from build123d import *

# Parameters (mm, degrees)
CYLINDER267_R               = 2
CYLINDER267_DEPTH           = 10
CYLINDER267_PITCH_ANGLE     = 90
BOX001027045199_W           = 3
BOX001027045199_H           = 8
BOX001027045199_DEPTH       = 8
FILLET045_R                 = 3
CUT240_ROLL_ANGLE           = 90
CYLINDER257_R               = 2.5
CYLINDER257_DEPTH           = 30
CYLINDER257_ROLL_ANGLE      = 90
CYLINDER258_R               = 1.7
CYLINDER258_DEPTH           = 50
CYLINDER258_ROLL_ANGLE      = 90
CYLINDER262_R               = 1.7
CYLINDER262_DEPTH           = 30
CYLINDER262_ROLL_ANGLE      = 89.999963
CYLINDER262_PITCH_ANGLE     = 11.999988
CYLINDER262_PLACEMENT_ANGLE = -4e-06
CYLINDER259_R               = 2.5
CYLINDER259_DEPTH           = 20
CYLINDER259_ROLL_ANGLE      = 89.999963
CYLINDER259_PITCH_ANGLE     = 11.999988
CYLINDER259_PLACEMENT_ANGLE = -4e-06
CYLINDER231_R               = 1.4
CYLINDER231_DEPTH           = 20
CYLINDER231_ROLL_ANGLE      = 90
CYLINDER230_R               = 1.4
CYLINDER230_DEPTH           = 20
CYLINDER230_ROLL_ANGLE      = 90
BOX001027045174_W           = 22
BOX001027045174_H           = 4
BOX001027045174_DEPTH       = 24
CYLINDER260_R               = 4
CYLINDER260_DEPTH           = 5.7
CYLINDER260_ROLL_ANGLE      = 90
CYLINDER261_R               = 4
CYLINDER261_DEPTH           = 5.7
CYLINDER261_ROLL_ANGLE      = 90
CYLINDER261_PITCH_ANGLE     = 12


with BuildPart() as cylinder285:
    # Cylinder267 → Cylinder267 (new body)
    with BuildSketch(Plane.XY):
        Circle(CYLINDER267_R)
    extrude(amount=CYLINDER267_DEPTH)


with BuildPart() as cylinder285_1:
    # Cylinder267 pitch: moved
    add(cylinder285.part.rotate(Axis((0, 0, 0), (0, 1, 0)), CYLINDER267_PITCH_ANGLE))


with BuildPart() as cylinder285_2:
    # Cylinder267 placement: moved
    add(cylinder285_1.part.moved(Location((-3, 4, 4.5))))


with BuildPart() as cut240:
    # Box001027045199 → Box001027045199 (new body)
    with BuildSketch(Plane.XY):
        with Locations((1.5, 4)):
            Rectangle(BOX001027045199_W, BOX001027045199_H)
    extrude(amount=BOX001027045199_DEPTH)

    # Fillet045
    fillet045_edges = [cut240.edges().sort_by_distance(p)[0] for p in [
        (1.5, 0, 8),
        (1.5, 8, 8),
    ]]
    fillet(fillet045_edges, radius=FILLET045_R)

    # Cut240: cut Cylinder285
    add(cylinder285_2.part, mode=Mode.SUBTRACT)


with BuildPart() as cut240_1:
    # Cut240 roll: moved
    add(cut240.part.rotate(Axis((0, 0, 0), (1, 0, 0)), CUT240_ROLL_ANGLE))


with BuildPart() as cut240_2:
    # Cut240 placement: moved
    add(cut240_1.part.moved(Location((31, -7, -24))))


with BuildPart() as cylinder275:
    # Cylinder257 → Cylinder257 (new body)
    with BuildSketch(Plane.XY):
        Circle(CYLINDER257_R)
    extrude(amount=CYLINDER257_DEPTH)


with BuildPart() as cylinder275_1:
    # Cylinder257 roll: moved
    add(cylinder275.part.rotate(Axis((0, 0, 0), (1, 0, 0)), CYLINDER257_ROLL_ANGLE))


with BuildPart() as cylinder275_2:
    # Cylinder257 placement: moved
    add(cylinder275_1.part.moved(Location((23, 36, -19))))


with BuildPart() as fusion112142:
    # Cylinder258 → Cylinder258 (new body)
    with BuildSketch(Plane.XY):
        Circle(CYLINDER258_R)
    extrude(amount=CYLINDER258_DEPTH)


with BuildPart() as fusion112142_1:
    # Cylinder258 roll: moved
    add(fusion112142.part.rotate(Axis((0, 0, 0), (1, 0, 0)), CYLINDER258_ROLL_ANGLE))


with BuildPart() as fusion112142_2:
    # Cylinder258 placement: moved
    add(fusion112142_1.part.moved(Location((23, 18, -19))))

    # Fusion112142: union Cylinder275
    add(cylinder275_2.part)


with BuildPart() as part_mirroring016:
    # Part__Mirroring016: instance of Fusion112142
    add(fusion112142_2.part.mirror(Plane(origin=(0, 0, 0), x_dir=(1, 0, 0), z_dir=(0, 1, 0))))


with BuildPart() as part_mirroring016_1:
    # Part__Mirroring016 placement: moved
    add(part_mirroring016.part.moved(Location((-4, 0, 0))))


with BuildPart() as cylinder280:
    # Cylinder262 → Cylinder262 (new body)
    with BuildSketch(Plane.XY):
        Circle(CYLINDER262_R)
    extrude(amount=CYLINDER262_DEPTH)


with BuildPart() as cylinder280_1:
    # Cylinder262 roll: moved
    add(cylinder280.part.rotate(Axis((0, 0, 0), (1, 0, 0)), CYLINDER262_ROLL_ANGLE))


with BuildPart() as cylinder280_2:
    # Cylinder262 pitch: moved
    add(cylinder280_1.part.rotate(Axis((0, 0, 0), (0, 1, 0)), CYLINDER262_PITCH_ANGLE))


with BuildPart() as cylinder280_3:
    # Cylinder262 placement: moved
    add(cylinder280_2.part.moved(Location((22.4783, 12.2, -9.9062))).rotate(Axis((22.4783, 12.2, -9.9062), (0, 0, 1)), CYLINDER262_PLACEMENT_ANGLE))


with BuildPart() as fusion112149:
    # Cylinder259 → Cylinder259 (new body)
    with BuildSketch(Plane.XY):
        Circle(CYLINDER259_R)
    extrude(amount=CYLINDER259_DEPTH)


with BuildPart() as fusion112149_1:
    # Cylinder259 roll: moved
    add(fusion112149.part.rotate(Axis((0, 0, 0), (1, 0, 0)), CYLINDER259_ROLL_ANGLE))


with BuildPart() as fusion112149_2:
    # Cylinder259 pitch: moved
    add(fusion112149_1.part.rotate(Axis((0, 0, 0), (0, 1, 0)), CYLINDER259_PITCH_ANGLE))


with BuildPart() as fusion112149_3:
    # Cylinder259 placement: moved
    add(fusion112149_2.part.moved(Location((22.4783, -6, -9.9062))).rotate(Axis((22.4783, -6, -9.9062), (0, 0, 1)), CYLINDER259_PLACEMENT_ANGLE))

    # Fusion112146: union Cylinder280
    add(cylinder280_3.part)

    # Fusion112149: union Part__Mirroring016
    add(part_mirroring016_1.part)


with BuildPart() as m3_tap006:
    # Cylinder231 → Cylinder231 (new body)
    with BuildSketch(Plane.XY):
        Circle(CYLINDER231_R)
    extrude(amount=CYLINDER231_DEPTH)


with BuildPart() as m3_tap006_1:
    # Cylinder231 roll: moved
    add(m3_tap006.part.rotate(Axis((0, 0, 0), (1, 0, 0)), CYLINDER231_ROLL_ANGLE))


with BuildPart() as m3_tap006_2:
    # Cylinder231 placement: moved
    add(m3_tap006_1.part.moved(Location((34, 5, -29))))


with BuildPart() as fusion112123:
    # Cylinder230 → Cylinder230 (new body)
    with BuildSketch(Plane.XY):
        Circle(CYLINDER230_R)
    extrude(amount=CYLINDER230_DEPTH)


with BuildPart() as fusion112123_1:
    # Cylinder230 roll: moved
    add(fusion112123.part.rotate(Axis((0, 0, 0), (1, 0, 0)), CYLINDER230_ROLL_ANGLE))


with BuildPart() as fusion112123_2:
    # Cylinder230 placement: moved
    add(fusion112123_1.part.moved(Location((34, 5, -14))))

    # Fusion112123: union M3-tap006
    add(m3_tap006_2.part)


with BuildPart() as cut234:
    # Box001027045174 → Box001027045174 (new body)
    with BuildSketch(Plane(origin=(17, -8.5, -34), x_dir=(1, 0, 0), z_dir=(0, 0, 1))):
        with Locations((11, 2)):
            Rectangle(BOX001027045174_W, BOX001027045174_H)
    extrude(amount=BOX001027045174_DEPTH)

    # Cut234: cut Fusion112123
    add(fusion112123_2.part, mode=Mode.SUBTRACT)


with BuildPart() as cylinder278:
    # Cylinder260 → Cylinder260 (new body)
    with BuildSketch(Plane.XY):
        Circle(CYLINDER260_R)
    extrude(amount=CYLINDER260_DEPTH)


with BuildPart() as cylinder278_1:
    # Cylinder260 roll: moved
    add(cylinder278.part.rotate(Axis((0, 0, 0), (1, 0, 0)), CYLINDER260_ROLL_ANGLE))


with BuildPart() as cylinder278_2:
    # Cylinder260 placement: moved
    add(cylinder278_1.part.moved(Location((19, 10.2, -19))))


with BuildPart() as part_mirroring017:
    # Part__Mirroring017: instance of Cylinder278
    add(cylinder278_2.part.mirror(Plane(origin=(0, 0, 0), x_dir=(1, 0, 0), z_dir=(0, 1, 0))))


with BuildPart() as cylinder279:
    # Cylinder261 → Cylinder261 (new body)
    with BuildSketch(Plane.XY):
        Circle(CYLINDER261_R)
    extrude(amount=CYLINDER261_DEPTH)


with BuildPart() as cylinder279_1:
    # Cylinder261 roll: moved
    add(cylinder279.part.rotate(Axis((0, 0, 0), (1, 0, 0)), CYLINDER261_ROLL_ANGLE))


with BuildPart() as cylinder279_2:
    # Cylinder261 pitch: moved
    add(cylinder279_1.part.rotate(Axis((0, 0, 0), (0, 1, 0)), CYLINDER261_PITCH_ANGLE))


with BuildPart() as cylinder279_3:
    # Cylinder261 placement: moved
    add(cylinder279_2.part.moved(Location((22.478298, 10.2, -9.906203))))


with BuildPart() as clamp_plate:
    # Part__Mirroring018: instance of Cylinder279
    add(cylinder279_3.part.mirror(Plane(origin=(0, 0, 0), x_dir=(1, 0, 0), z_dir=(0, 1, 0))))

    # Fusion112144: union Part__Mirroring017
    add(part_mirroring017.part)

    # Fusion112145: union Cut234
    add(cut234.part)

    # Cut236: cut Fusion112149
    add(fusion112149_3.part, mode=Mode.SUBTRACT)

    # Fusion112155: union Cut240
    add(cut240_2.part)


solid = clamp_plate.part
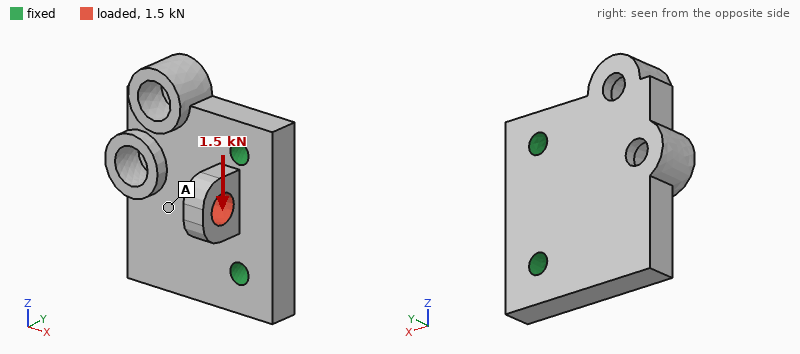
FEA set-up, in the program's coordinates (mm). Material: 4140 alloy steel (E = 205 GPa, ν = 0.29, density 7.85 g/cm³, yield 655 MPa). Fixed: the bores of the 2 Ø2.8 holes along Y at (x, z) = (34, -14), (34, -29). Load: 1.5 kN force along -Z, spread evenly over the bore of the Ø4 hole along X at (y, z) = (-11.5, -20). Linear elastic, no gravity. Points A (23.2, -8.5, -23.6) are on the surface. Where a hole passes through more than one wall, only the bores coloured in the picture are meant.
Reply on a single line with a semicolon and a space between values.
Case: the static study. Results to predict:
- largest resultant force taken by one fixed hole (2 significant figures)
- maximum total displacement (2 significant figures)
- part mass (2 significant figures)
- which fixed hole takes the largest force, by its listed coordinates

1.1 kN; 16 µm; 18 g; (34, -14)
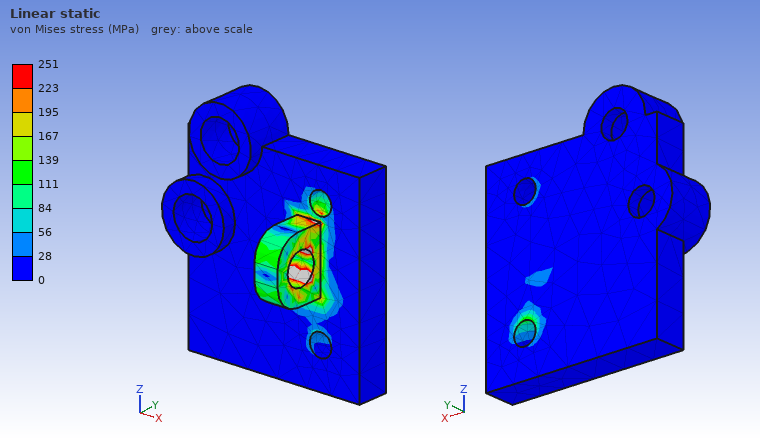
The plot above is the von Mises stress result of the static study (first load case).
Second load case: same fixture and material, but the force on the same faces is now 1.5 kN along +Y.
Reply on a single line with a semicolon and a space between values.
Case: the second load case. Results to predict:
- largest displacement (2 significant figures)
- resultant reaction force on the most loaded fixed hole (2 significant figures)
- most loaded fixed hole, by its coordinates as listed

6.3 µm; 930 N; (34, -14)
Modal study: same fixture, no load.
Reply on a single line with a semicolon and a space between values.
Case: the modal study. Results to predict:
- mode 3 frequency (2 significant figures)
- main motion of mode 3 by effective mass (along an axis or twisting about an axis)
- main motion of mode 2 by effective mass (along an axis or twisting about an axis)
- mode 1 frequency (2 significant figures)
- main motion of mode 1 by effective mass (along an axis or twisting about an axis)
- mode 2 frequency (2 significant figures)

30 kHz; along Z; twisting about X; 9900 Hz; along Y; 17 kHz
